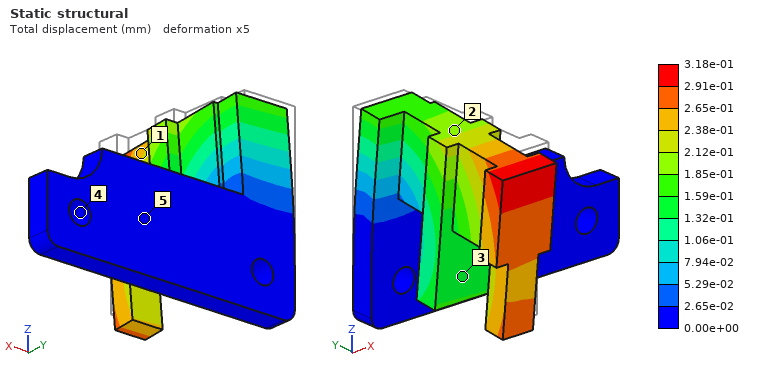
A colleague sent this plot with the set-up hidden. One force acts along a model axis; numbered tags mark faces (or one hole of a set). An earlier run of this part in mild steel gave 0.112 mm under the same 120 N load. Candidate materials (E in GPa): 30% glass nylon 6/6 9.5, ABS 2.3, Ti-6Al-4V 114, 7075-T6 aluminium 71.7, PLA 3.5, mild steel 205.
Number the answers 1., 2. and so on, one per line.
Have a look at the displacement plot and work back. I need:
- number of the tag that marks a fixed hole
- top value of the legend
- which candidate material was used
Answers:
1. 4
2. 3.18e-01 mm
3. 7075-T6 aluminium
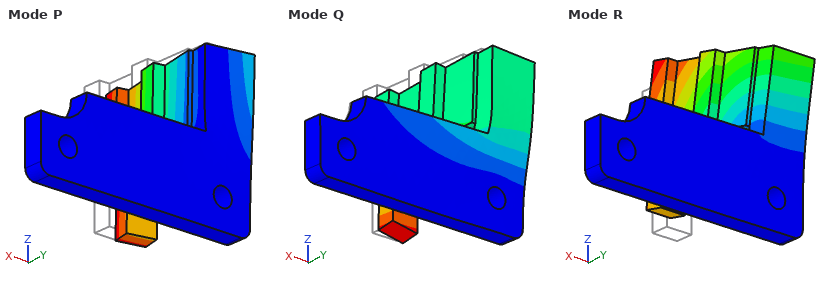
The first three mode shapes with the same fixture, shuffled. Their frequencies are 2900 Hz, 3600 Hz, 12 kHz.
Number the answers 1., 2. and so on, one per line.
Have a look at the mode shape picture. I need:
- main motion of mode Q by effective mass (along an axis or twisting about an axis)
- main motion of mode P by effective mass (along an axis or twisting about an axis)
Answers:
1. along Y
2. along X
